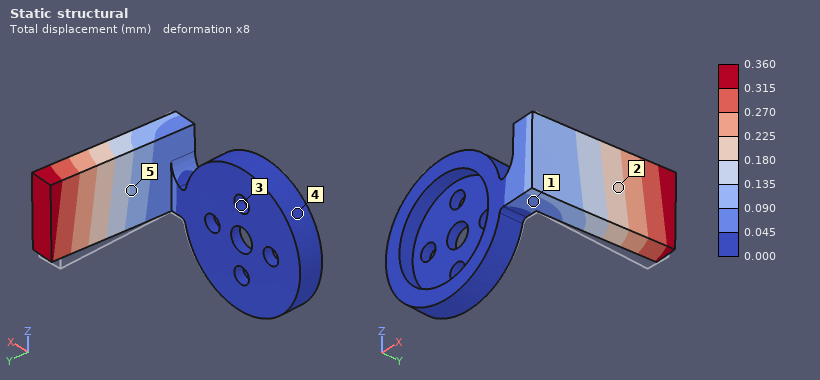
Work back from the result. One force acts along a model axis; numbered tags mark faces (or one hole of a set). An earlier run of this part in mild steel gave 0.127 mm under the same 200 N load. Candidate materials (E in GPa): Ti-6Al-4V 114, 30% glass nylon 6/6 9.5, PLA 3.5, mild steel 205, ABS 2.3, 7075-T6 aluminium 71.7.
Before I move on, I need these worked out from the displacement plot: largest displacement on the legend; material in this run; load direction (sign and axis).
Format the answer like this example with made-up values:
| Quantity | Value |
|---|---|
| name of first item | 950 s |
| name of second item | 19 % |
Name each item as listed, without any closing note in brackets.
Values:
| Quantity | Value |
|---|---|
| largest displacement on the legend | 0.360 mm |
| material in this run | 7075-T6 aluminium |
| load direction | +X |
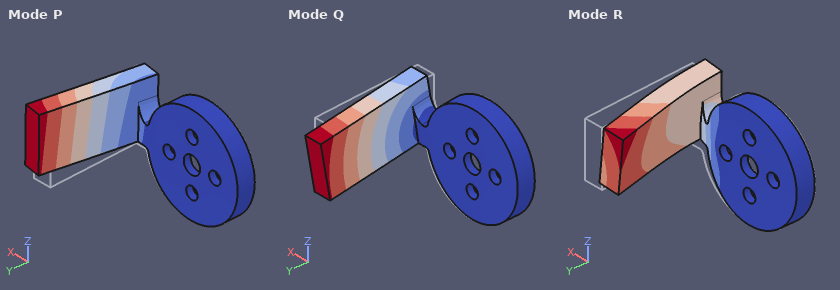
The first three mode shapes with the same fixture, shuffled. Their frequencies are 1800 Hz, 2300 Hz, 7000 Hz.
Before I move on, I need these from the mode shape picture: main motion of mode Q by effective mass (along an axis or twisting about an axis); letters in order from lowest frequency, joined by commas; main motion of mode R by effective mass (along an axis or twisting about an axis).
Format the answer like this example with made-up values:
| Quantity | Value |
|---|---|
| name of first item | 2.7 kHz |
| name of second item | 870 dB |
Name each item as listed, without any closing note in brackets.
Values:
| Quantity | Value |
|---|---|
| main motion of mode Q by effective mass | along Z |
| letters in order from lowest frequency, joined by commas | P, Q, R |
| main motion of mode R by effective mass | along Y |
